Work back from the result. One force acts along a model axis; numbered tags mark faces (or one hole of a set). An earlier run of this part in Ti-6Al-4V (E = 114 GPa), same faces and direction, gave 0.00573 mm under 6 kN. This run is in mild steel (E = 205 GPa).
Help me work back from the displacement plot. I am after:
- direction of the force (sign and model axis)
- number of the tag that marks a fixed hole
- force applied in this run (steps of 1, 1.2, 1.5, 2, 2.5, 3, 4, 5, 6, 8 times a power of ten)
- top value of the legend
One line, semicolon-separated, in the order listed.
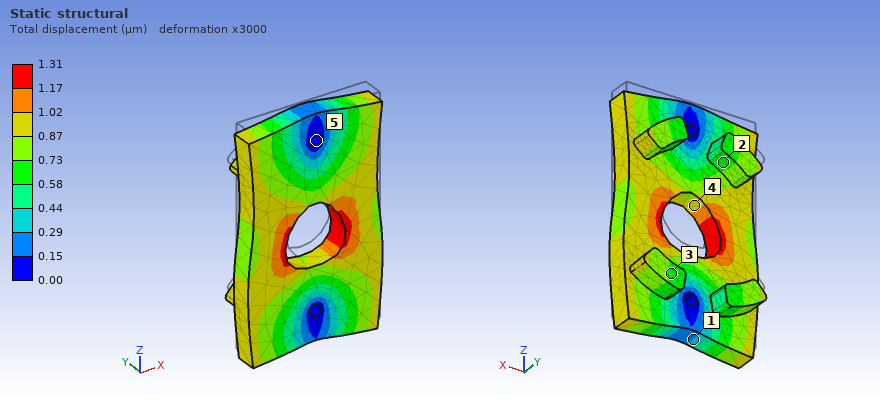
-Z; 5; 2.5 kN; 1.31 µm
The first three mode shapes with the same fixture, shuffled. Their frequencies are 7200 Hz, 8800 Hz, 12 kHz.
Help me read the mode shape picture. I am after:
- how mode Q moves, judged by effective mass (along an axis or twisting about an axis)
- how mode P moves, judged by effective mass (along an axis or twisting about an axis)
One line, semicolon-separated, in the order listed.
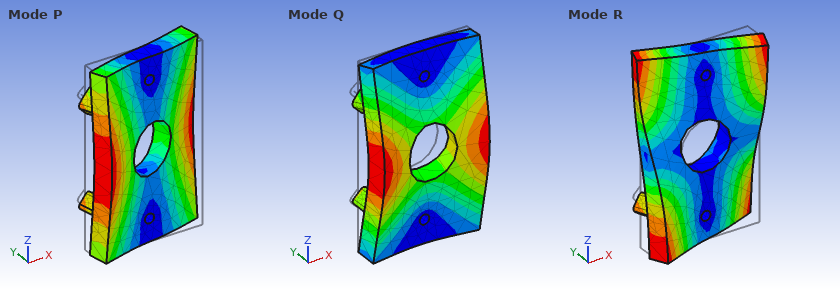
along Y; twisting about Z
